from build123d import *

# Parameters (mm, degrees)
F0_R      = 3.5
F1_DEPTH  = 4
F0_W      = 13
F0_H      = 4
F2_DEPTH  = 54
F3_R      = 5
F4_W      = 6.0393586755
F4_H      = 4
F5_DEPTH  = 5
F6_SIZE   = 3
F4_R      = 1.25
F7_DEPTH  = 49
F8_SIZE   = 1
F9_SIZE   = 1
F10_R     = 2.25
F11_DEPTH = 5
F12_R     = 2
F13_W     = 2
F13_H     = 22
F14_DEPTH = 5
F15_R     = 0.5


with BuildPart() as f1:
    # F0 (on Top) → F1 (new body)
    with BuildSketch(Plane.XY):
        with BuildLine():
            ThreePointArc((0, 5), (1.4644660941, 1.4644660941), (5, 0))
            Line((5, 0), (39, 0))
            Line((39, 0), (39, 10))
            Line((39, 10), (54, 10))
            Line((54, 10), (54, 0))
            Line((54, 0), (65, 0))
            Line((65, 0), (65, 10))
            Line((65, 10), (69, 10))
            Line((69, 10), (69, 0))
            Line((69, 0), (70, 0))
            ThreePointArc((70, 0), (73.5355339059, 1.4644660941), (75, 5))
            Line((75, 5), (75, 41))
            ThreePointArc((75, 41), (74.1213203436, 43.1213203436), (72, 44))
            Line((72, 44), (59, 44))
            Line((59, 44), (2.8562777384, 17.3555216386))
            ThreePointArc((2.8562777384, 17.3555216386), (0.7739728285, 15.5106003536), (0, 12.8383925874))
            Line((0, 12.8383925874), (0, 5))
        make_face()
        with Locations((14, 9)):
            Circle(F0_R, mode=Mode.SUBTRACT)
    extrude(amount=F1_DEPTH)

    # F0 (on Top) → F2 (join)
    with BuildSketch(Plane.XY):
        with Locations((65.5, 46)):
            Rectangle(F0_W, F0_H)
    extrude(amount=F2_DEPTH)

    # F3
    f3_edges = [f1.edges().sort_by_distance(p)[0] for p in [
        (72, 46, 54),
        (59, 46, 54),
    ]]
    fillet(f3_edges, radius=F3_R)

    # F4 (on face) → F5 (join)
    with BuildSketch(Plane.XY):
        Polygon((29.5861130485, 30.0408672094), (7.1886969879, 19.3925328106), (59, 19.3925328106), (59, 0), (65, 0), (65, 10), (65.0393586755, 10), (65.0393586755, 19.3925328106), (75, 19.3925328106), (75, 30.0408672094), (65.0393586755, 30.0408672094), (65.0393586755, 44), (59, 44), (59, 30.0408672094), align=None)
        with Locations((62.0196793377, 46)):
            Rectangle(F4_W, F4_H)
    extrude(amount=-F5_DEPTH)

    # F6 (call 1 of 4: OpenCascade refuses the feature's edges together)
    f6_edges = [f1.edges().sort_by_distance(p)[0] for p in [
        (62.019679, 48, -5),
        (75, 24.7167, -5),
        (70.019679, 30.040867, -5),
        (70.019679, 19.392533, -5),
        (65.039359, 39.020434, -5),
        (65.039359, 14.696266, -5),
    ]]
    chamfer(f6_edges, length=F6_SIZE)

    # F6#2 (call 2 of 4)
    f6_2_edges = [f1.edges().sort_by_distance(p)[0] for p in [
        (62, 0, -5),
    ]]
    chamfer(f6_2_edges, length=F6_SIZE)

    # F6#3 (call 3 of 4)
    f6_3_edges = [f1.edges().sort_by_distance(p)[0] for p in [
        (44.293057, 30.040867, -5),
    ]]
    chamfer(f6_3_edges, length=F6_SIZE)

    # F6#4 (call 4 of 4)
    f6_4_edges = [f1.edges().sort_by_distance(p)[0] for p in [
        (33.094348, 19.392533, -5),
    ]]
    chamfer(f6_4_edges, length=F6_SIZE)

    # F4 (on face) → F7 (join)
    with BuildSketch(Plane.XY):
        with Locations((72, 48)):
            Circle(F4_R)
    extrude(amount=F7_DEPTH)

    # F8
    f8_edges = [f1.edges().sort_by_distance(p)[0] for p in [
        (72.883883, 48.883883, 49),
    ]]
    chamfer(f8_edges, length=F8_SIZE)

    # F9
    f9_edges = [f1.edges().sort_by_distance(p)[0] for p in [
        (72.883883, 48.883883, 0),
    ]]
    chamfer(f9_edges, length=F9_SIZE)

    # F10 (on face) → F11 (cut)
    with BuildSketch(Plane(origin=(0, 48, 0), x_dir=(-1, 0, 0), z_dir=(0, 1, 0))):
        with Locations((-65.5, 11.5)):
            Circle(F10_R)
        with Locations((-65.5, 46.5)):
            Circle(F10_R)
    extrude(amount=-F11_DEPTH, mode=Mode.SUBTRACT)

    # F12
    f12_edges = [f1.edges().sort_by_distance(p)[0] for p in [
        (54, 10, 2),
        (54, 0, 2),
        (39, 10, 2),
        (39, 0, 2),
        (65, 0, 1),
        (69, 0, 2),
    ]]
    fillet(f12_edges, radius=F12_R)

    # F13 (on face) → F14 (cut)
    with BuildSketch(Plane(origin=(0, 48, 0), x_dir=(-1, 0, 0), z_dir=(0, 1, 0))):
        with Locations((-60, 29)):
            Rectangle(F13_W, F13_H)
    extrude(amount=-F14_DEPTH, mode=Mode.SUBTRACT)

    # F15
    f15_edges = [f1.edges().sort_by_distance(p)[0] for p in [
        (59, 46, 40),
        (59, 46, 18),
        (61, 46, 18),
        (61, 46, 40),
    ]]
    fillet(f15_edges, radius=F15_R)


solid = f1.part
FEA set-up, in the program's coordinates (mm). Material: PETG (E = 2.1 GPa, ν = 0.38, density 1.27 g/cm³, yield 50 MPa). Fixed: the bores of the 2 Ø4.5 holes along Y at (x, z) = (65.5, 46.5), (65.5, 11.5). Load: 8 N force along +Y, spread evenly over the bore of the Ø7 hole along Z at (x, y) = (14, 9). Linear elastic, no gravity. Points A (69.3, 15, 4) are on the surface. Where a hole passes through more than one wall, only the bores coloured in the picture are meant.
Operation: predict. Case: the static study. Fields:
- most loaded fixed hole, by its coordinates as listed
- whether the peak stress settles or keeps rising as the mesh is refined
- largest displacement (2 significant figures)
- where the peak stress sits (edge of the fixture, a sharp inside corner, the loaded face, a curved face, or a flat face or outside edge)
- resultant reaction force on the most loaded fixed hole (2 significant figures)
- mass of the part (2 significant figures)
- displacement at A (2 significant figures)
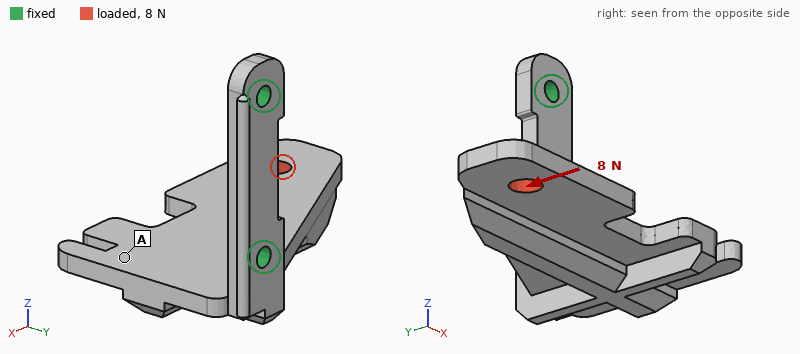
(65.5, 11.5)
keeps rising
1.2 mm
edge of the fixture
7.7 N
19 g
0.45 mm
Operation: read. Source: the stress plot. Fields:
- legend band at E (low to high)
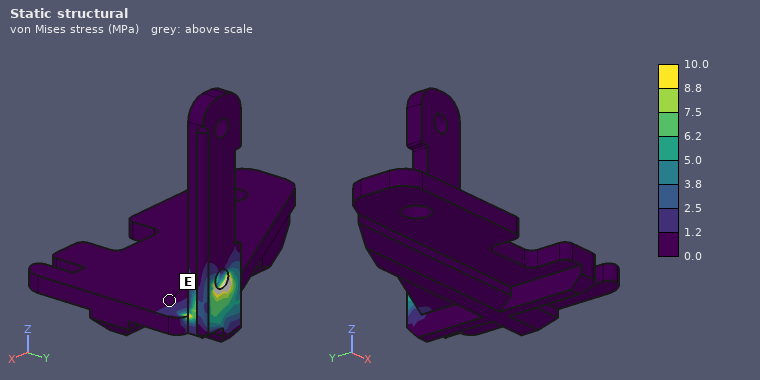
0.0 to 1.2 MPa
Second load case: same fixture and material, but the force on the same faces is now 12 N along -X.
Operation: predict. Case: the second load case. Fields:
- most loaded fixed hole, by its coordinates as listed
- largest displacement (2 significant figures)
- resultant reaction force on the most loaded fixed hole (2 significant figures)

(65.5, 11.5)
1.2 mm
14 N
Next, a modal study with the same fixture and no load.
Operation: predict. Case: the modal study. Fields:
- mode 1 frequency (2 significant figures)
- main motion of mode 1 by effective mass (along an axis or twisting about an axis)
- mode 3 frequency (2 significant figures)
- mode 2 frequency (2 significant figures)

140 Hz
along Z
400 Hz
180 Hz
